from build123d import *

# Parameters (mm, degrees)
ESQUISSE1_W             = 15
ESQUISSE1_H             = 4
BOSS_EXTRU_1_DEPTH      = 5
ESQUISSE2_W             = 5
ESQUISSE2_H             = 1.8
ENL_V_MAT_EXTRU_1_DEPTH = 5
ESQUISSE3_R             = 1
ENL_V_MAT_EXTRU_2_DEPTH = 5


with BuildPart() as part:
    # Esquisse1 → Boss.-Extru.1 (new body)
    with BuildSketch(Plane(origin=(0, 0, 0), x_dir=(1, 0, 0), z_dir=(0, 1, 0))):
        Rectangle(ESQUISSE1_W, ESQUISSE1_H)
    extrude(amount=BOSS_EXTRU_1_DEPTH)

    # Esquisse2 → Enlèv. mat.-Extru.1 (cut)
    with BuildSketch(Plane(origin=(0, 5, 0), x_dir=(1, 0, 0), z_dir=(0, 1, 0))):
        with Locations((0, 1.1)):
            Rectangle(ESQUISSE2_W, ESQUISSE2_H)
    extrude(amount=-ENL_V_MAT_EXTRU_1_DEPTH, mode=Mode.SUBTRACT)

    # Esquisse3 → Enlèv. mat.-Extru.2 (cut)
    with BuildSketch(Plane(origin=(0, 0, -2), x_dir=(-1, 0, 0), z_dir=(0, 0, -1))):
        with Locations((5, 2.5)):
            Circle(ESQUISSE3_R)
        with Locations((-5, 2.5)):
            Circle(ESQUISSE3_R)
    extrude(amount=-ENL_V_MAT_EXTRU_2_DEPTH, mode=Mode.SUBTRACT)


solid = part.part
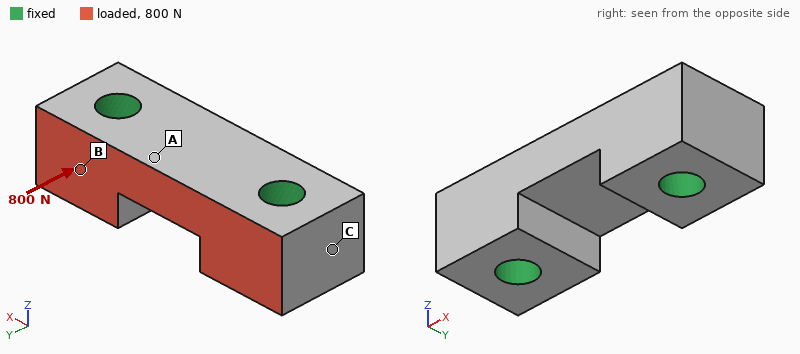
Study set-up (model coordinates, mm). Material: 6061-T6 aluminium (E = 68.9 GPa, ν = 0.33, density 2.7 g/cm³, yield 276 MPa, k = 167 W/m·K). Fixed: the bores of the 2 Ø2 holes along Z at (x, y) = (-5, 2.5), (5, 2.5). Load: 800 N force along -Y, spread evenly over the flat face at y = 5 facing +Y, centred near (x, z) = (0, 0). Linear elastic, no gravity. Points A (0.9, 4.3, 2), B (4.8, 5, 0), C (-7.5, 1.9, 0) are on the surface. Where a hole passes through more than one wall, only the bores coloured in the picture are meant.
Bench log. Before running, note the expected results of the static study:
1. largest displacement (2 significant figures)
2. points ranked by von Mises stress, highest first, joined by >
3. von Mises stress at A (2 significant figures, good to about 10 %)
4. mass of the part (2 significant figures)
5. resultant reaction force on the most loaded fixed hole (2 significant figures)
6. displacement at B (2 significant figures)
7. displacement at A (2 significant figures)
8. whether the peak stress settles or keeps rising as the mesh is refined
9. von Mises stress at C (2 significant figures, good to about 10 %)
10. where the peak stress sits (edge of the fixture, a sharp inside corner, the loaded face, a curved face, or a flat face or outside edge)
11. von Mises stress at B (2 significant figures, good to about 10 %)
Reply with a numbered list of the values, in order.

1. 2.3 µm
2. B > A > C
3. 15 MPa
4. 0.62 g
5. 400 N
6. 0.51 µm
7. 2.1 µm
8. keeps rising
9. 7.1 MPa
10. edge of the fixture
11. 29 MPa
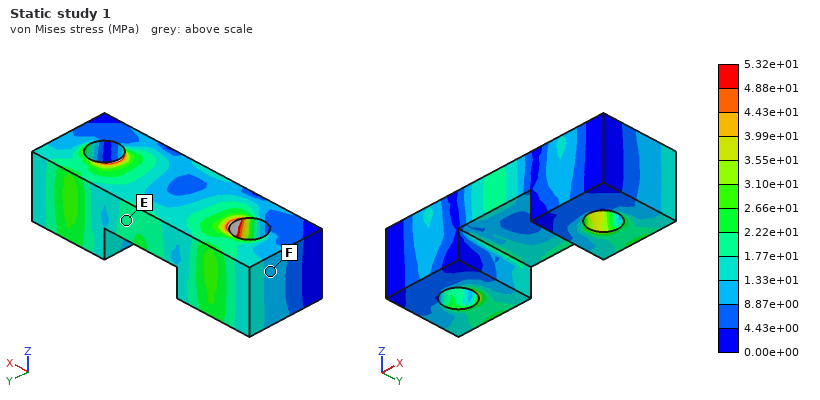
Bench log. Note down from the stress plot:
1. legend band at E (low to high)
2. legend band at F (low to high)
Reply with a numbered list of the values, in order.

1. 1.77e+01 to 2.22e+01 MPa
2. 8.87e+00 to 1.33e+01 MPa
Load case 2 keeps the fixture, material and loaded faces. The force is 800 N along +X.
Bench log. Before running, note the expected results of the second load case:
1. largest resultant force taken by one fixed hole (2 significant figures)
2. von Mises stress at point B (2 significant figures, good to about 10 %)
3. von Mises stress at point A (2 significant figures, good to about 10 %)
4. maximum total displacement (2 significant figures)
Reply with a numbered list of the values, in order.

1. 410 N
2. 29 MPa
3. 25 MPa
4. 3.0 µm
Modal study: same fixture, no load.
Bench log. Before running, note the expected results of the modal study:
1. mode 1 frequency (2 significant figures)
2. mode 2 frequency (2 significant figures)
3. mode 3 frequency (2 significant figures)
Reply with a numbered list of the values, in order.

1. 140 kHz
2. 140 kHz
3. 170 kHz
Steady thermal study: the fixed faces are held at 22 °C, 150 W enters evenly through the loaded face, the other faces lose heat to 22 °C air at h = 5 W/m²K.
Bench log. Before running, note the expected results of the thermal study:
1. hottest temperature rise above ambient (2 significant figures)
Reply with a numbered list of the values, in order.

1. 65 K
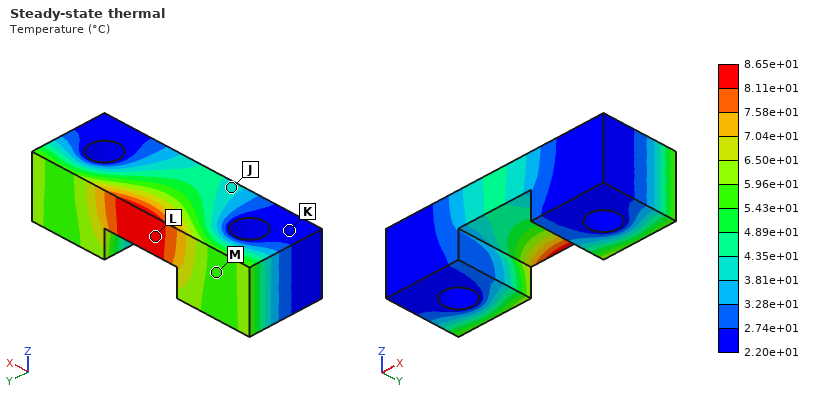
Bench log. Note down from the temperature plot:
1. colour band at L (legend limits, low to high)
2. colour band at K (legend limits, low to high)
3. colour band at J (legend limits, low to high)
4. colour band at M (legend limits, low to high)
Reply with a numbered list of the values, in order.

1. 8.11e+01 to 8.65e+01 °C
2. 2.20e+01 to 2.74e+01 °C
3. 3.81e+01 to 4.35e+01 °C
4. 5.43e+01 to 5.96e+01 °C
